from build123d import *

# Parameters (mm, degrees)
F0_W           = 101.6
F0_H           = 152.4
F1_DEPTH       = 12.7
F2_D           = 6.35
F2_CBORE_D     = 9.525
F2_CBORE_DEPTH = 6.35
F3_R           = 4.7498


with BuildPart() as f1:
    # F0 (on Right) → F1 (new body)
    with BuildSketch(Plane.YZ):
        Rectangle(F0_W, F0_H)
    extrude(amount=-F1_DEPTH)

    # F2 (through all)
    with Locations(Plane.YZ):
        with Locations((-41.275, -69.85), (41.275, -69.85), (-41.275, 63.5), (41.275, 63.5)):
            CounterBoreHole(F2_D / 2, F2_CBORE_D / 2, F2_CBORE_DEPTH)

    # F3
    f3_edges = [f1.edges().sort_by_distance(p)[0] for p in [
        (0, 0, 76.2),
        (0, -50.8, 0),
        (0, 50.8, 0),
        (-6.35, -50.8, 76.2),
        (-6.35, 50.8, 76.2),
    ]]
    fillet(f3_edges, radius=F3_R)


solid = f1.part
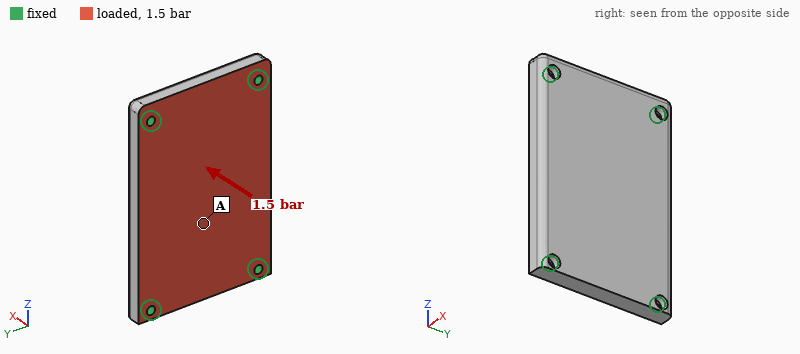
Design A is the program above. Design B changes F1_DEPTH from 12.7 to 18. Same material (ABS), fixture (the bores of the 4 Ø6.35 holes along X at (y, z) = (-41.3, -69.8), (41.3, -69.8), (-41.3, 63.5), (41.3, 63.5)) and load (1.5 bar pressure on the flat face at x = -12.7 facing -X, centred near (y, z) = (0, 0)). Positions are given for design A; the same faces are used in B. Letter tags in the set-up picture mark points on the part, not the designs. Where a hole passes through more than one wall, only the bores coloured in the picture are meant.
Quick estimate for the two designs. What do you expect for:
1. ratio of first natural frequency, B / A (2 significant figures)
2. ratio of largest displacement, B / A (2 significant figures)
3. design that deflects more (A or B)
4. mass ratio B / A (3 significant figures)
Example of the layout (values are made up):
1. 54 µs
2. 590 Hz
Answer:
1. 1.4
2. 0.37
3. A
4. 1.42
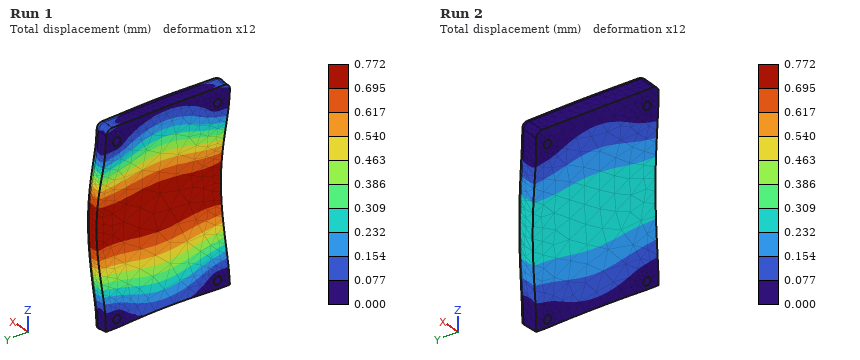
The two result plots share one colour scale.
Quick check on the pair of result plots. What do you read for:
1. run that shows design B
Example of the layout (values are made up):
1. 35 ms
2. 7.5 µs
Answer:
1. Run 2
